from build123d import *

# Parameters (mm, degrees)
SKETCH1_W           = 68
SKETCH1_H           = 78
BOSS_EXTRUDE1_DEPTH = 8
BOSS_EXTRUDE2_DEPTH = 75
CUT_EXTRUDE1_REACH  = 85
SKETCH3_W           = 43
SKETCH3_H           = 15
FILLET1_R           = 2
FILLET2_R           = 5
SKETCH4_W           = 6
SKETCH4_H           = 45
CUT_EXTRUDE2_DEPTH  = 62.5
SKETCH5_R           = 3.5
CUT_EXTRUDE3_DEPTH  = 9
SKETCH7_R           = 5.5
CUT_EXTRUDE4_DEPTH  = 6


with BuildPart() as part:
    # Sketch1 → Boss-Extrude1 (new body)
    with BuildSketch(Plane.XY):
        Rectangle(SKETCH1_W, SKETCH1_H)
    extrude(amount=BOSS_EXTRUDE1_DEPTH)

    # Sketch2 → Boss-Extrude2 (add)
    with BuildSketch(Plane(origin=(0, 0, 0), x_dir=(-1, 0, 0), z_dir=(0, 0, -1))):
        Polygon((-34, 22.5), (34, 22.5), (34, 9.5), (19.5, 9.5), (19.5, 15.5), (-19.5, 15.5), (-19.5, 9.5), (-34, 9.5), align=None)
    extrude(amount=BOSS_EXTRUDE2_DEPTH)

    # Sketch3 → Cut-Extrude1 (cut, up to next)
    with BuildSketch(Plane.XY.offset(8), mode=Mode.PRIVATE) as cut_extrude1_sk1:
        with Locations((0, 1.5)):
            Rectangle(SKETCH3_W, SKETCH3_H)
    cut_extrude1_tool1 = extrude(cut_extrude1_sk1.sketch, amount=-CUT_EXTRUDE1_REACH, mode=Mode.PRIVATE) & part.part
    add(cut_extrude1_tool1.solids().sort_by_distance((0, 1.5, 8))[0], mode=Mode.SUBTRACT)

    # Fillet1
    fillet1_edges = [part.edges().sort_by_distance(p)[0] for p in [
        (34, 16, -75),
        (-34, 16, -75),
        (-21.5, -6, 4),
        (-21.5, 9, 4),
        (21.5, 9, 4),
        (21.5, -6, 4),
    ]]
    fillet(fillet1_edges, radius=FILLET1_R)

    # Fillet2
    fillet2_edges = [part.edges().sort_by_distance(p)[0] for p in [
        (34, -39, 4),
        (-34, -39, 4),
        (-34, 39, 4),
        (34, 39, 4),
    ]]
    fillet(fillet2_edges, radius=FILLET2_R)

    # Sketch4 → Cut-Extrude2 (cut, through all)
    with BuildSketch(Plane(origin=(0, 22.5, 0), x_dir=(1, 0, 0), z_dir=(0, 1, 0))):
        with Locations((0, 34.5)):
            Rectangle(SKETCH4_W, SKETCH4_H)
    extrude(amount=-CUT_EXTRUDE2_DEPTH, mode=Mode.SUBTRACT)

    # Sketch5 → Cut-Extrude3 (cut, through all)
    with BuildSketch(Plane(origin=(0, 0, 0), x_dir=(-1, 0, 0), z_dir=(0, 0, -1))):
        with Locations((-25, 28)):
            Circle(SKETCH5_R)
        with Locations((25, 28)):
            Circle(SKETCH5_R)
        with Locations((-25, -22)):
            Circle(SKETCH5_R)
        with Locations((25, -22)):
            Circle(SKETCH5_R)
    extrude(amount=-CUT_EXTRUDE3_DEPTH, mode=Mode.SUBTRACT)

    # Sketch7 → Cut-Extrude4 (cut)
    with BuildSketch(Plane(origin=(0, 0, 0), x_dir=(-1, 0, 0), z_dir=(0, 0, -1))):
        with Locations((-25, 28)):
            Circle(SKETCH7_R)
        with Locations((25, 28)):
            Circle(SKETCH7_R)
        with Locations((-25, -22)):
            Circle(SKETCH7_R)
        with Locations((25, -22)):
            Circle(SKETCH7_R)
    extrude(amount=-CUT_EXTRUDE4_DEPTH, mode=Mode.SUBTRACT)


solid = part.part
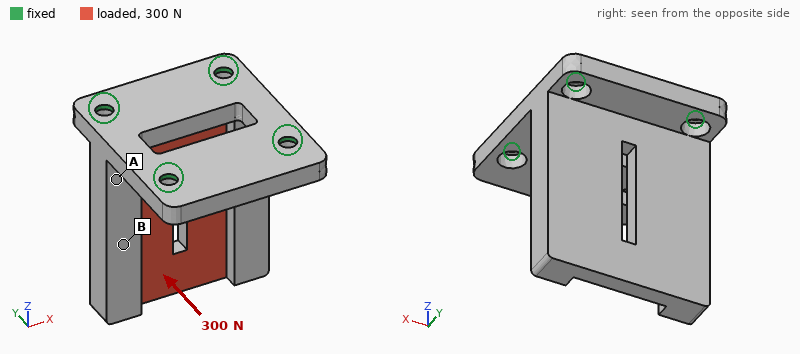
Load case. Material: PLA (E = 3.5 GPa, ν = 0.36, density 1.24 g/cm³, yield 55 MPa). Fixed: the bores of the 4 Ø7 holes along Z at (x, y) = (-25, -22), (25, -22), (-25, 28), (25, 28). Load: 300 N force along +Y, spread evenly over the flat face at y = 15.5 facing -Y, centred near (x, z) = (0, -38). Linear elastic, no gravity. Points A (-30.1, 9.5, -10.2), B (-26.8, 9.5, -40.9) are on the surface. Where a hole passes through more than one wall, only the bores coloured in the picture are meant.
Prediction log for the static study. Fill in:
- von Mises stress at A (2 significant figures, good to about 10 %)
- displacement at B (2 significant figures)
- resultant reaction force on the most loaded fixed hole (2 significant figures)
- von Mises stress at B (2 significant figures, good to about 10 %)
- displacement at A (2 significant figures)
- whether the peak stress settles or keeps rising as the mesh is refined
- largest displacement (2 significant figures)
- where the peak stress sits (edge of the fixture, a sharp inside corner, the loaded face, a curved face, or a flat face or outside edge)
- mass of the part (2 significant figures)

8.1 MPa
0.78 mm
310 N
2.8 MPa
0.25 mm
keeps rising
1.6 mm
edge of the fixture
100 g
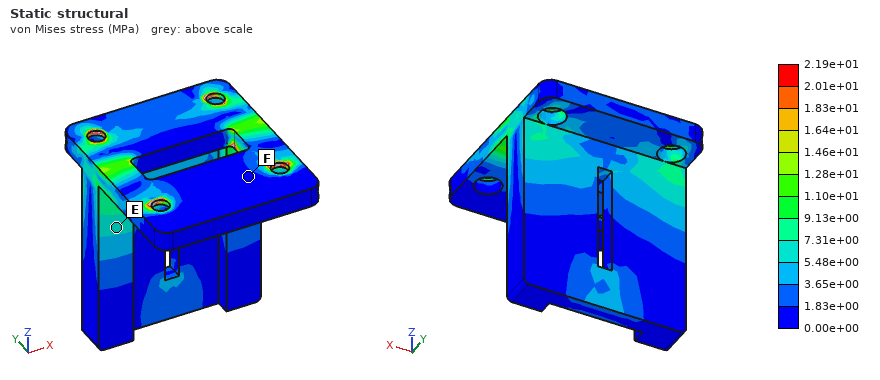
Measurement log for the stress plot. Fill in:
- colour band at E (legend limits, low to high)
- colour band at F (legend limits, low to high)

5.48e+00 to 7.31e+00 MPa
0.00e+00 to 1.83e+00 MPa
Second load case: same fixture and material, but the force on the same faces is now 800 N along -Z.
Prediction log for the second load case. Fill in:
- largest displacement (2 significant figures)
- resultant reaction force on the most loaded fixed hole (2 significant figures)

0.56 mm
370 N
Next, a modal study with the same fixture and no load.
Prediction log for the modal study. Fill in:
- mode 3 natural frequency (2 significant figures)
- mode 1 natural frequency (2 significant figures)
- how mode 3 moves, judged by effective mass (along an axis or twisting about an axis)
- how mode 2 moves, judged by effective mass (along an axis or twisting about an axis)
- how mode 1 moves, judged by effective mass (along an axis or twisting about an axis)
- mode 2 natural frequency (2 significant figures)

950 Hz
360 Hz
along X
twisting about Z
along Y
850 Hz
